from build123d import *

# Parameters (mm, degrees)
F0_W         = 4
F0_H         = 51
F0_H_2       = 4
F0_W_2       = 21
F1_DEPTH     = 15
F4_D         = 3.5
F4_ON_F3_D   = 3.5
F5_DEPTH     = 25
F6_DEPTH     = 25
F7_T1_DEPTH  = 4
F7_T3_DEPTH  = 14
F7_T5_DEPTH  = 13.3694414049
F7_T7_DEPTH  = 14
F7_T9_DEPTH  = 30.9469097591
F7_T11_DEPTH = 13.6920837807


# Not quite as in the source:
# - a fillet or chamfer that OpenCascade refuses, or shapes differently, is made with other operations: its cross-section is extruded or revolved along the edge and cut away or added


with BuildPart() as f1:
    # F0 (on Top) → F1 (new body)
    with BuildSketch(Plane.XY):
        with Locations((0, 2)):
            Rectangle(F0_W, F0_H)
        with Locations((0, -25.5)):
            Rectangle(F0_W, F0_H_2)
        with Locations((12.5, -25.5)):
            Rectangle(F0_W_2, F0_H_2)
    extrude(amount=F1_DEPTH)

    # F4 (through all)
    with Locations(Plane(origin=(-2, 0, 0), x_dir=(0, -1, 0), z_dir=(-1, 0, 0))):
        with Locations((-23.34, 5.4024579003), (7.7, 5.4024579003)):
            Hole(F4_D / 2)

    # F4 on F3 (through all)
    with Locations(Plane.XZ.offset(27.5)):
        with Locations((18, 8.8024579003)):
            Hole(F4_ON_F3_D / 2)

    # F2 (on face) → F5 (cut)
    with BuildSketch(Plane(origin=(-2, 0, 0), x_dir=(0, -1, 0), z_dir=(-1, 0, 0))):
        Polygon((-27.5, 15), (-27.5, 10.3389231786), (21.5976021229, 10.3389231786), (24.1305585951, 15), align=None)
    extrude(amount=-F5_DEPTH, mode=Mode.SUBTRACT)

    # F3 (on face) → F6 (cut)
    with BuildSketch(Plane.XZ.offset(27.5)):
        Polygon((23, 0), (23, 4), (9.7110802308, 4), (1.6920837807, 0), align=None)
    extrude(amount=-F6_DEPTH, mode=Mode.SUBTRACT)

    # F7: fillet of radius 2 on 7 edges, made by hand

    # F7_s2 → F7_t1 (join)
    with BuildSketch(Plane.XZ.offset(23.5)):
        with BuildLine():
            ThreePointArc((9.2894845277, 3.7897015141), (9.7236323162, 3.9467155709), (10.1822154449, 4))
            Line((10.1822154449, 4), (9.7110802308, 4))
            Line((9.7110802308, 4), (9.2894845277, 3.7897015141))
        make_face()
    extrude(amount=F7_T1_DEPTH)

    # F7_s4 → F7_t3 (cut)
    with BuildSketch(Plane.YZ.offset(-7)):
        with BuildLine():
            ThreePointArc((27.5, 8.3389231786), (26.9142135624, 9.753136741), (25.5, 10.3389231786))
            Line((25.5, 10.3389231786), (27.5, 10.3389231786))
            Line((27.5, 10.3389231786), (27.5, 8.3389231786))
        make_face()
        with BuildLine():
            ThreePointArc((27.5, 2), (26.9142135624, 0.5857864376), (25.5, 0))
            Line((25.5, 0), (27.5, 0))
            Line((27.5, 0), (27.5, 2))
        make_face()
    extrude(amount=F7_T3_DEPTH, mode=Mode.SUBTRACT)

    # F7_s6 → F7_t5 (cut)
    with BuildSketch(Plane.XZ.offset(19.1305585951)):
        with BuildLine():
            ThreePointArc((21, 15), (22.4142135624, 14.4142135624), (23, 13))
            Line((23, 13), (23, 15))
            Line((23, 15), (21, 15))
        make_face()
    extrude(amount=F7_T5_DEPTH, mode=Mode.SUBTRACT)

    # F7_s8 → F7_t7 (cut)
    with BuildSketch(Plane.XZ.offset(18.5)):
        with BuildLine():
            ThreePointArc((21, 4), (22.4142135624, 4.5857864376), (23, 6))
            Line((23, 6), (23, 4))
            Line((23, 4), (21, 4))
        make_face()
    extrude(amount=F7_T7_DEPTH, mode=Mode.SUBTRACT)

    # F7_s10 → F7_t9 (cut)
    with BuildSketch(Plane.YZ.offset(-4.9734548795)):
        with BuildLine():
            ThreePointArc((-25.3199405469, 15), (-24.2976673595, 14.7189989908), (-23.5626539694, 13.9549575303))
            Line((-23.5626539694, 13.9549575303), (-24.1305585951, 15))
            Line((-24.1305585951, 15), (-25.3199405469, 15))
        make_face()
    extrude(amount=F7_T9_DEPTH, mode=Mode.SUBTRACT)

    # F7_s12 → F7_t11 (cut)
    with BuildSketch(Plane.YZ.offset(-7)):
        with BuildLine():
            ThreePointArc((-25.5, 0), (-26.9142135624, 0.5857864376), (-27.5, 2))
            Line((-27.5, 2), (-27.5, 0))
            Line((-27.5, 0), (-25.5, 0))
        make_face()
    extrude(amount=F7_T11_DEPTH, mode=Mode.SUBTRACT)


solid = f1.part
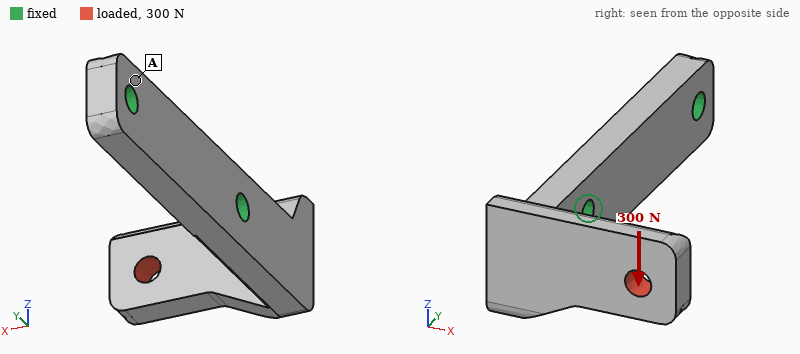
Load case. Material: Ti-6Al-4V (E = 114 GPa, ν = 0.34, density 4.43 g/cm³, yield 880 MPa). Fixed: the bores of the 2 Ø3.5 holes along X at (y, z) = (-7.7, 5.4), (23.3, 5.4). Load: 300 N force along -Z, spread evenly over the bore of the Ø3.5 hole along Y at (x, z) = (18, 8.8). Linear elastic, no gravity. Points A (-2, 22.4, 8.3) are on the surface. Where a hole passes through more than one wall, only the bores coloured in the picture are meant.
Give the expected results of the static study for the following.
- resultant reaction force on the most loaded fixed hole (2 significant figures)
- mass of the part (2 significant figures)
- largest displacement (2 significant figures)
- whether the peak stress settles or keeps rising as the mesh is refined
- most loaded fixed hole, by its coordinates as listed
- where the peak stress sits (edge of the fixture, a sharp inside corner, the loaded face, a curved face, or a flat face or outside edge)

370 N
14 g
0.31 mm
keeps rising
(-7.7, 5.4)
edge of the fixture
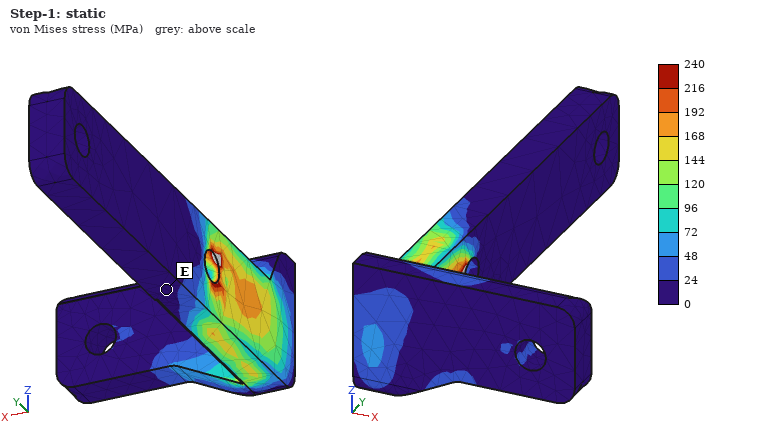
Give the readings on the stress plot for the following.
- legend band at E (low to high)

0 to 24 MPa
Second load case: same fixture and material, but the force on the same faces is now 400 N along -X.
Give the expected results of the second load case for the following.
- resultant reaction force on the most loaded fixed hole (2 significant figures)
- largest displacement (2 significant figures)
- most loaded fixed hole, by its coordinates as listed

410 N
0.27 mm
(-7.7, 5.4)
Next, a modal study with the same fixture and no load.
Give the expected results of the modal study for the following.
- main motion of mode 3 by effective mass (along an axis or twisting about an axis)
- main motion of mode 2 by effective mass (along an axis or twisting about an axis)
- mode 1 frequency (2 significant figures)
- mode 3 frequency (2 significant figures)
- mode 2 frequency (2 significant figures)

along X
along Z
2700 Hz
7800 Hz
3600 Hz
